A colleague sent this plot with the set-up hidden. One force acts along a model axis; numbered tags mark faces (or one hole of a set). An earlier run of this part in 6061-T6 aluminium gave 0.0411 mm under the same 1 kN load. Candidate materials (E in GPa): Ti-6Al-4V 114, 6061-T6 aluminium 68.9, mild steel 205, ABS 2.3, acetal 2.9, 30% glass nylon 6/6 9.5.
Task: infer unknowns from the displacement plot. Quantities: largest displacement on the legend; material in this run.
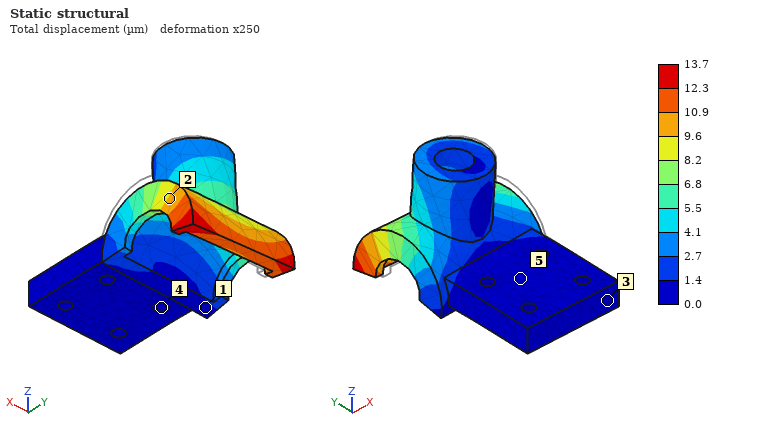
13.7 µm
mild steel
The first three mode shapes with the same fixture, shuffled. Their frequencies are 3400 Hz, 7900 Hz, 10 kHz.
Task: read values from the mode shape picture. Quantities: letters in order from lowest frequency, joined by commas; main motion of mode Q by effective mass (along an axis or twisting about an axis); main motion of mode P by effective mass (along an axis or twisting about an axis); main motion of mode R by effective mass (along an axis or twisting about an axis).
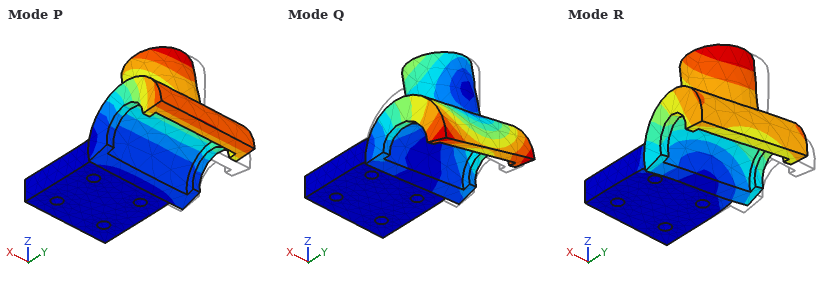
P, Q, R
twisting about Y
along Z
along X
